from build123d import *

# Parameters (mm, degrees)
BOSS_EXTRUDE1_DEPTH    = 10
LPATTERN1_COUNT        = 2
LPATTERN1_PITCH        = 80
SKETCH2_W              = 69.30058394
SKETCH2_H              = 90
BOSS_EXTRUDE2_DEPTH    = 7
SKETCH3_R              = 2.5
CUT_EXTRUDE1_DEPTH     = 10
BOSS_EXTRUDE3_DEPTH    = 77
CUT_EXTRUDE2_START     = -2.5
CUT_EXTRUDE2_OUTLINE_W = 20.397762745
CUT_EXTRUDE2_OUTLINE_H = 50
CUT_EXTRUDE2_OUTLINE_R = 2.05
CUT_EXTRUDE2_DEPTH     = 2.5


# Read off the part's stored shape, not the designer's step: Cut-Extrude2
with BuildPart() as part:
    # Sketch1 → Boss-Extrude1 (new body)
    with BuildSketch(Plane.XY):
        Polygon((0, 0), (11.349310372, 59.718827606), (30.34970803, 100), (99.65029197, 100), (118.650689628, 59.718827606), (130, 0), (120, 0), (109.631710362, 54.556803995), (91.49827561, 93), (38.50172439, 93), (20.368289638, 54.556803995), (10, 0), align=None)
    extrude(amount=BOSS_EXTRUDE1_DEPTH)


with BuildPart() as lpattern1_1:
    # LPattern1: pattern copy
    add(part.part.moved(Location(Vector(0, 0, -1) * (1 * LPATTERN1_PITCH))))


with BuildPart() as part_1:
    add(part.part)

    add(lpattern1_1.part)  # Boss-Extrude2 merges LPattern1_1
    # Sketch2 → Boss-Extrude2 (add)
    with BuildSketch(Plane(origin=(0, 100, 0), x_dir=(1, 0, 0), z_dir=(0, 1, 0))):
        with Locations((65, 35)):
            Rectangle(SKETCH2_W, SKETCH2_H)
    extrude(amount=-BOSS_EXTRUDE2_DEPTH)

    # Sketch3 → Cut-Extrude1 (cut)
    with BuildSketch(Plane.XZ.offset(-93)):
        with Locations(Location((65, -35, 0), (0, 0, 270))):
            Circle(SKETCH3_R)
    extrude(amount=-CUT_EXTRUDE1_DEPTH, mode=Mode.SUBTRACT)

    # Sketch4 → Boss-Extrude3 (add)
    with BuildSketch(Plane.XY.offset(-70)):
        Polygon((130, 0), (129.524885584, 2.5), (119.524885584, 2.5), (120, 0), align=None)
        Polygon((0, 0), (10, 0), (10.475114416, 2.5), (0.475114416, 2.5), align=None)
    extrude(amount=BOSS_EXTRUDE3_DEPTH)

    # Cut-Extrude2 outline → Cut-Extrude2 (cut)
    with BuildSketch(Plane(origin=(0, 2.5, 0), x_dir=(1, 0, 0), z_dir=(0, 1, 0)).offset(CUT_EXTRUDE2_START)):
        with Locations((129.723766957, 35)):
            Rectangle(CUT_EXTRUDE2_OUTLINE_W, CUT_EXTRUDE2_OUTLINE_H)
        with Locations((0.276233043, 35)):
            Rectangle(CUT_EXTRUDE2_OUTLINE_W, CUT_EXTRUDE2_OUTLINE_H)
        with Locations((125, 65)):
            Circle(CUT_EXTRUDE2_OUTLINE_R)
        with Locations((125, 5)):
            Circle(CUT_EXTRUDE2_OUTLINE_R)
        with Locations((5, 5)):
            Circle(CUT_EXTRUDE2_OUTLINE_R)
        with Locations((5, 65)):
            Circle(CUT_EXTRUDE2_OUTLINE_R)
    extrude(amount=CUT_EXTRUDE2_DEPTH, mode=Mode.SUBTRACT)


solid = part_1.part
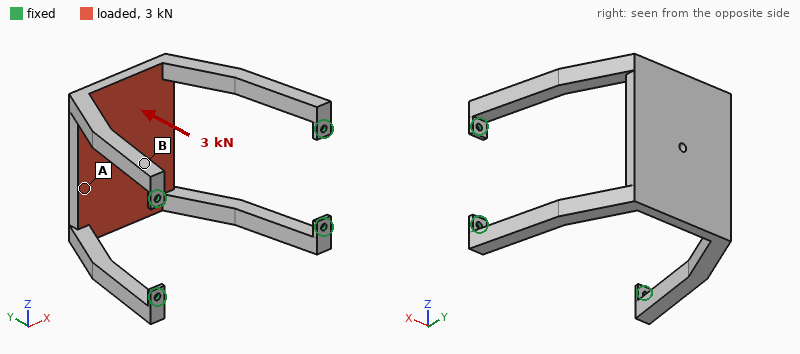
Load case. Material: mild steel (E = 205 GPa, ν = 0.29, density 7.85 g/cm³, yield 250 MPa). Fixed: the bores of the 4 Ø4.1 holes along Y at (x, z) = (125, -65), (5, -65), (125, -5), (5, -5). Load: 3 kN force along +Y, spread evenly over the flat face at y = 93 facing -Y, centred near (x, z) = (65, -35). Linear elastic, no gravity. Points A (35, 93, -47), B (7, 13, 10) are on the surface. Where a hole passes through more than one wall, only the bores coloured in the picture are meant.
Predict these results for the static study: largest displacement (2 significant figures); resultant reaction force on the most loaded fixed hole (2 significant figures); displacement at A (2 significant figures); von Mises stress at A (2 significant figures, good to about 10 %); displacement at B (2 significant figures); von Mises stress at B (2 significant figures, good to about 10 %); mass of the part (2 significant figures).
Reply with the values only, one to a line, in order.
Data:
64 µm
790 N
53 µm
36 MPa
22 µm
17 MPa
660 g
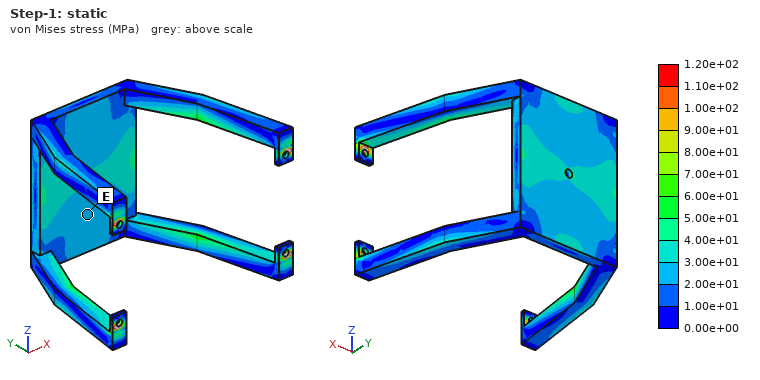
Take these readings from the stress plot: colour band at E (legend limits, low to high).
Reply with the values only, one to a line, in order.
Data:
2.00e+01 to 3.00e+01 MPa
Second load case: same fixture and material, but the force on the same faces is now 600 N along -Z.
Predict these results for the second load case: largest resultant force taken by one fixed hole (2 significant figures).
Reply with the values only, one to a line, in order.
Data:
360 N
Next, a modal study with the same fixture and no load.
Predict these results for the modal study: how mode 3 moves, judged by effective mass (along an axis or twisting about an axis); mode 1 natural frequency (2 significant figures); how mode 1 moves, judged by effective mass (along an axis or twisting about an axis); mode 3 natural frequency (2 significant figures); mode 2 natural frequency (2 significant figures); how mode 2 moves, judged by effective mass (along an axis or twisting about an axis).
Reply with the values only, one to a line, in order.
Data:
twisting about Y
260 Hz
along Z
780 Hz
540 Hz
along X
